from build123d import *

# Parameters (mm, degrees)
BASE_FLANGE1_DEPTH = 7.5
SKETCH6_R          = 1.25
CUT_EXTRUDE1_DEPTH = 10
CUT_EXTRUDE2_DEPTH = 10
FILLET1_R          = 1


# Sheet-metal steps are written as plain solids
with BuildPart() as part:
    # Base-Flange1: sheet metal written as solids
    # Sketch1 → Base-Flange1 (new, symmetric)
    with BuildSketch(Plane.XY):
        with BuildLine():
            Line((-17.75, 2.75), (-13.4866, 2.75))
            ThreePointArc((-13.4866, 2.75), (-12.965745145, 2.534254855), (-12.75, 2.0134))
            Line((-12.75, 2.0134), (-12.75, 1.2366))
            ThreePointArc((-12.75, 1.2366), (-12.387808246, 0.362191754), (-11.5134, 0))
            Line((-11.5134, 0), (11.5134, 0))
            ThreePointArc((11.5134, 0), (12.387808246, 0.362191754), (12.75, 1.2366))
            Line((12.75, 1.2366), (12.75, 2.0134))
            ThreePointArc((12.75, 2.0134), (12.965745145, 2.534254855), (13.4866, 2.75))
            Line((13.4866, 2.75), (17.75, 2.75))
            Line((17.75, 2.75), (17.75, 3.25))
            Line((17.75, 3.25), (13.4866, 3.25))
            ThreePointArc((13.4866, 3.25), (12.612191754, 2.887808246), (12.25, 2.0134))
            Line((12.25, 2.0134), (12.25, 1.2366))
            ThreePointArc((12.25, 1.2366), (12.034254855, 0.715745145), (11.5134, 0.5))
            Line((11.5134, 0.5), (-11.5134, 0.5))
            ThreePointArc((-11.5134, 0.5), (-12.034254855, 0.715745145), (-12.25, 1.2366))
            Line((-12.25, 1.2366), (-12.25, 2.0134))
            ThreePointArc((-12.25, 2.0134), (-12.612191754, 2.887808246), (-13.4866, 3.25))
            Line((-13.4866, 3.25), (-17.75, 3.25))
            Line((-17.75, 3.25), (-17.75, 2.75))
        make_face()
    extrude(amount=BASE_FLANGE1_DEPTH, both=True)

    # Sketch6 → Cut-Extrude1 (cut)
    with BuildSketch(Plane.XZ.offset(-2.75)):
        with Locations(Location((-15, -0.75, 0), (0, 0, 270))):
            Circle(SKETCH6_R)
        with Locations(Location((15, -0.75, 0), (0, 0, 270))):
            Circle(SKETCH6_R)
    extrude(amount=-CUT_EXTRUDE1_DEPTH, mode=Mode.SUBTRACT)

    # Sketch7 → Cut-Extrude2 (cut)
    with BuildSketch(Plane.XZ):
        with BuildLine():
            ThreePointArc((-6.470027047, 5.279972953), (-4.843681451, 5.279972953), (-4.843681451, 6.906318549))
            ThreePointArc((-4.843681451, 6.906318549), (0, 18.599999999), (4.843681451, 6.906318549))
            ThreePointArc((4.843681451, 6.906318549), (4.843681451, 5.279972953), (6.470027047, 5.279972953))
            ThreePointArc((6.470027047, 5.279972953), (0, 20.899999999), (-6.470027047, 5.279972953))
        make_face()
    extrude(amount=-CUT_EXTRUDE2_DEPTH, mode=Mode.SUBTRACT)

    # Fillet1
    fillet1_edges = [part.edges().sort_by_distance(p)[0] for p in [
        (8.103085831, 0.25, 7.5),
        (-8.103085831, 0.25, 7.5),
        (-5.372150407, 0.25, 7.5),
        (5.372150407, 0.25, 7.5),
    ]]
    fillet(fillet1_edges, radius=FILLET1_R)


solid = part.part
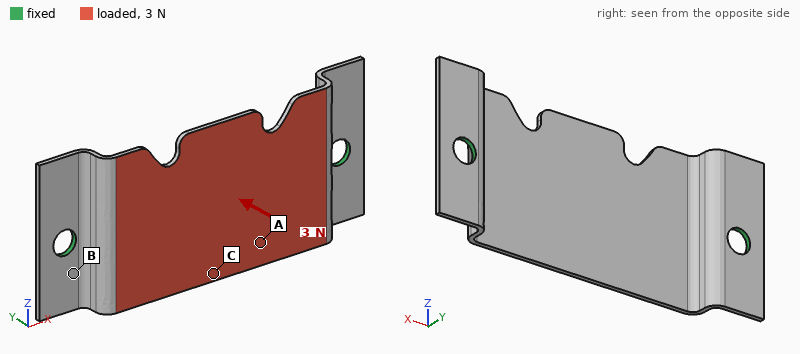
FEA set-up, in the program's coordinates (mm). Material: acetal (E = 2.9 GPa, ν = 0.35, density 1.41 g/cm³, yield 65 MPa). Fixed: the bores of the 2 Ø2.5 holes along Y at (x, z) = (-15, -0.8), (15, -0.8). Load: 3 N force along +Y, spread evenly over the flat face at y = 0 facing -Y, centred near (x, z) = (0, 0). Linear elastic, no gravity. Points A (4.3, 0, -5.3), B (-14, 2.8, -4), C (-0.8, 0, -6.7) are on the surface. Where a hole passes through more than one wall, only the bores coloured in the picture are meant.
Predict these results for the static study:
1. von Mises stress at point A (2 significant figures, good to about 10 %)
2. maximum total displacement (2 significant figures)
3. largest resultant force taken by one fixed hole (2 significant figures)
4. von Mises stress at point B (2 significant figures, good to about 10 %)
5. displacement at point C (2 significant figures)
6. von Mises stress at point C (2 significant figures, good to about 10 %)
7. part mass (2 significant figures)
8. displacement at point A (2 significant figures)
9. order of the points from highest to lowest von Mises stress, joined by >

4.0 MPa
0.37 mm
3.5 N
1.5 MPa
0.31 mm
6.0 MPa
0.40 g
0.24 mm
C > A > B
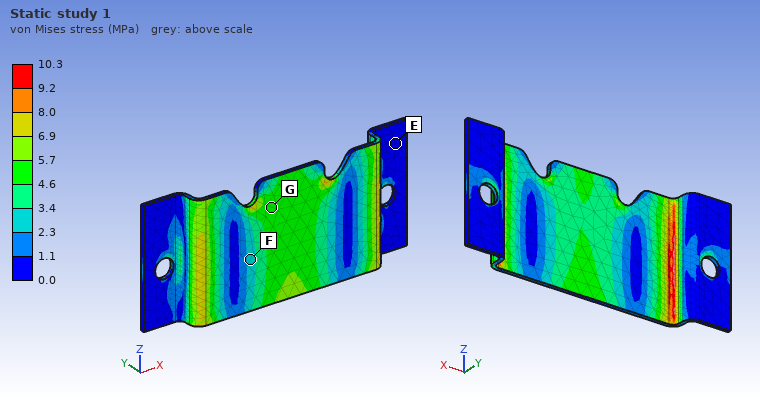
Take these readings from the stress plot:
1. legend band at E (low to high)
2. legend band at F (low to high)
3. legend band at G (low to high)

0.0 to 1.1 MPa
2.3 to 3.4 MPa
4.6 to 5.7 MPa
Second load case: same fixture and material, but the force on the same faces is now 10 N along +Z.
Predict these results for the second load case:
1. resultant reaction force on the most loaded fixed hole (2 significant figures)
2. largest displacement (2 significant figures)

5.0 N
0.24 mm
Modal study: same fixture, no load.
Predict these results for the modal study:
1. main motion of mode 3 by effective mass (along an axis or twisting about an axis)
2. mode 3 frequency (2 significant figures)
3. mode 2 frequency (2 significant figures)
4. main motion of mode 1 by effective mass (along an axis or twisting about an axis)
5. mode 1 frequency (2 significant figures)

along X
1900 Hz
1400 Hz
along Y
1100 Hz
